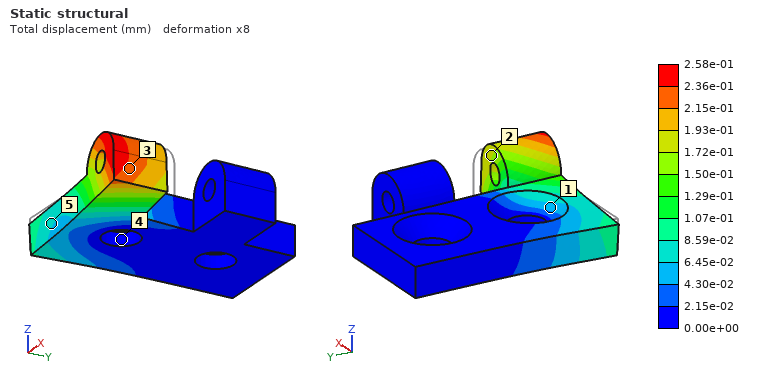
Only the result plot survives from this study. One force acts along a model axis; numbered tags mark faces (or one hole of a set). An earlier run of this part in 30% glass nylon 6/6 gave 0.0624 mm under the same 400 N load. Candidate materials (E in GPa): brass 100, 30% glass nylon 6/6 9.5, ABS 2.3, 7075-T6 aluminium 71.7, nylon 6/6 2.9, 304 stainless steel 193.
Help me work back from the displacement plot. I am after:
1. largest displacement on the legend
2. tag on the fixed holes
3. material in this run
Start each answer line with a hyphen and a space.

- 2.58e-01 mm
- 4
- ABS
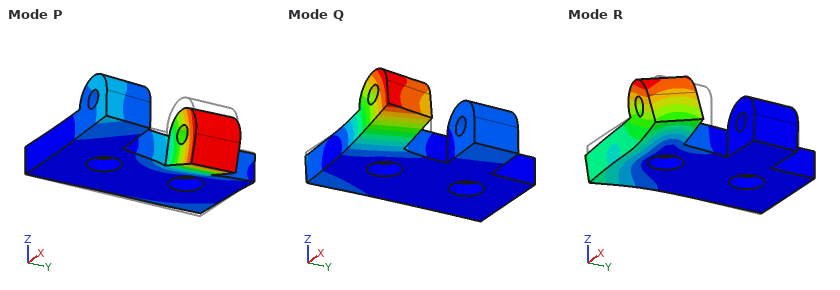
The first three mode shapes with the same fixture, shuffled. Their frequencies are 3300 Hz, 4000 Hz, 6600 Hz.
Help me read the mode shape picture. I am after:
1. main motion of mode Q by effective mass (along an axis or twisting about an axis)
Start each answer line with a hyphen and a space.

- along Z
